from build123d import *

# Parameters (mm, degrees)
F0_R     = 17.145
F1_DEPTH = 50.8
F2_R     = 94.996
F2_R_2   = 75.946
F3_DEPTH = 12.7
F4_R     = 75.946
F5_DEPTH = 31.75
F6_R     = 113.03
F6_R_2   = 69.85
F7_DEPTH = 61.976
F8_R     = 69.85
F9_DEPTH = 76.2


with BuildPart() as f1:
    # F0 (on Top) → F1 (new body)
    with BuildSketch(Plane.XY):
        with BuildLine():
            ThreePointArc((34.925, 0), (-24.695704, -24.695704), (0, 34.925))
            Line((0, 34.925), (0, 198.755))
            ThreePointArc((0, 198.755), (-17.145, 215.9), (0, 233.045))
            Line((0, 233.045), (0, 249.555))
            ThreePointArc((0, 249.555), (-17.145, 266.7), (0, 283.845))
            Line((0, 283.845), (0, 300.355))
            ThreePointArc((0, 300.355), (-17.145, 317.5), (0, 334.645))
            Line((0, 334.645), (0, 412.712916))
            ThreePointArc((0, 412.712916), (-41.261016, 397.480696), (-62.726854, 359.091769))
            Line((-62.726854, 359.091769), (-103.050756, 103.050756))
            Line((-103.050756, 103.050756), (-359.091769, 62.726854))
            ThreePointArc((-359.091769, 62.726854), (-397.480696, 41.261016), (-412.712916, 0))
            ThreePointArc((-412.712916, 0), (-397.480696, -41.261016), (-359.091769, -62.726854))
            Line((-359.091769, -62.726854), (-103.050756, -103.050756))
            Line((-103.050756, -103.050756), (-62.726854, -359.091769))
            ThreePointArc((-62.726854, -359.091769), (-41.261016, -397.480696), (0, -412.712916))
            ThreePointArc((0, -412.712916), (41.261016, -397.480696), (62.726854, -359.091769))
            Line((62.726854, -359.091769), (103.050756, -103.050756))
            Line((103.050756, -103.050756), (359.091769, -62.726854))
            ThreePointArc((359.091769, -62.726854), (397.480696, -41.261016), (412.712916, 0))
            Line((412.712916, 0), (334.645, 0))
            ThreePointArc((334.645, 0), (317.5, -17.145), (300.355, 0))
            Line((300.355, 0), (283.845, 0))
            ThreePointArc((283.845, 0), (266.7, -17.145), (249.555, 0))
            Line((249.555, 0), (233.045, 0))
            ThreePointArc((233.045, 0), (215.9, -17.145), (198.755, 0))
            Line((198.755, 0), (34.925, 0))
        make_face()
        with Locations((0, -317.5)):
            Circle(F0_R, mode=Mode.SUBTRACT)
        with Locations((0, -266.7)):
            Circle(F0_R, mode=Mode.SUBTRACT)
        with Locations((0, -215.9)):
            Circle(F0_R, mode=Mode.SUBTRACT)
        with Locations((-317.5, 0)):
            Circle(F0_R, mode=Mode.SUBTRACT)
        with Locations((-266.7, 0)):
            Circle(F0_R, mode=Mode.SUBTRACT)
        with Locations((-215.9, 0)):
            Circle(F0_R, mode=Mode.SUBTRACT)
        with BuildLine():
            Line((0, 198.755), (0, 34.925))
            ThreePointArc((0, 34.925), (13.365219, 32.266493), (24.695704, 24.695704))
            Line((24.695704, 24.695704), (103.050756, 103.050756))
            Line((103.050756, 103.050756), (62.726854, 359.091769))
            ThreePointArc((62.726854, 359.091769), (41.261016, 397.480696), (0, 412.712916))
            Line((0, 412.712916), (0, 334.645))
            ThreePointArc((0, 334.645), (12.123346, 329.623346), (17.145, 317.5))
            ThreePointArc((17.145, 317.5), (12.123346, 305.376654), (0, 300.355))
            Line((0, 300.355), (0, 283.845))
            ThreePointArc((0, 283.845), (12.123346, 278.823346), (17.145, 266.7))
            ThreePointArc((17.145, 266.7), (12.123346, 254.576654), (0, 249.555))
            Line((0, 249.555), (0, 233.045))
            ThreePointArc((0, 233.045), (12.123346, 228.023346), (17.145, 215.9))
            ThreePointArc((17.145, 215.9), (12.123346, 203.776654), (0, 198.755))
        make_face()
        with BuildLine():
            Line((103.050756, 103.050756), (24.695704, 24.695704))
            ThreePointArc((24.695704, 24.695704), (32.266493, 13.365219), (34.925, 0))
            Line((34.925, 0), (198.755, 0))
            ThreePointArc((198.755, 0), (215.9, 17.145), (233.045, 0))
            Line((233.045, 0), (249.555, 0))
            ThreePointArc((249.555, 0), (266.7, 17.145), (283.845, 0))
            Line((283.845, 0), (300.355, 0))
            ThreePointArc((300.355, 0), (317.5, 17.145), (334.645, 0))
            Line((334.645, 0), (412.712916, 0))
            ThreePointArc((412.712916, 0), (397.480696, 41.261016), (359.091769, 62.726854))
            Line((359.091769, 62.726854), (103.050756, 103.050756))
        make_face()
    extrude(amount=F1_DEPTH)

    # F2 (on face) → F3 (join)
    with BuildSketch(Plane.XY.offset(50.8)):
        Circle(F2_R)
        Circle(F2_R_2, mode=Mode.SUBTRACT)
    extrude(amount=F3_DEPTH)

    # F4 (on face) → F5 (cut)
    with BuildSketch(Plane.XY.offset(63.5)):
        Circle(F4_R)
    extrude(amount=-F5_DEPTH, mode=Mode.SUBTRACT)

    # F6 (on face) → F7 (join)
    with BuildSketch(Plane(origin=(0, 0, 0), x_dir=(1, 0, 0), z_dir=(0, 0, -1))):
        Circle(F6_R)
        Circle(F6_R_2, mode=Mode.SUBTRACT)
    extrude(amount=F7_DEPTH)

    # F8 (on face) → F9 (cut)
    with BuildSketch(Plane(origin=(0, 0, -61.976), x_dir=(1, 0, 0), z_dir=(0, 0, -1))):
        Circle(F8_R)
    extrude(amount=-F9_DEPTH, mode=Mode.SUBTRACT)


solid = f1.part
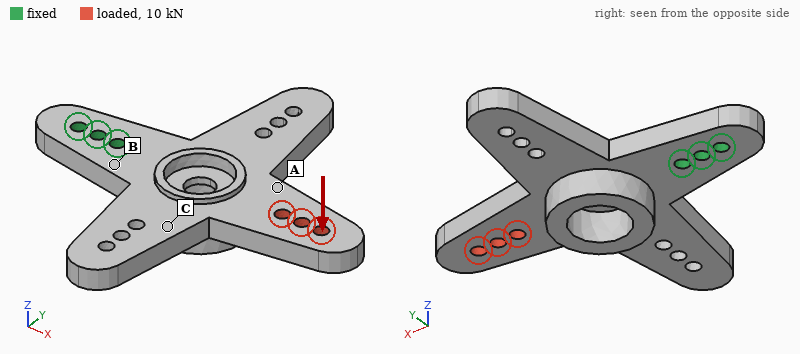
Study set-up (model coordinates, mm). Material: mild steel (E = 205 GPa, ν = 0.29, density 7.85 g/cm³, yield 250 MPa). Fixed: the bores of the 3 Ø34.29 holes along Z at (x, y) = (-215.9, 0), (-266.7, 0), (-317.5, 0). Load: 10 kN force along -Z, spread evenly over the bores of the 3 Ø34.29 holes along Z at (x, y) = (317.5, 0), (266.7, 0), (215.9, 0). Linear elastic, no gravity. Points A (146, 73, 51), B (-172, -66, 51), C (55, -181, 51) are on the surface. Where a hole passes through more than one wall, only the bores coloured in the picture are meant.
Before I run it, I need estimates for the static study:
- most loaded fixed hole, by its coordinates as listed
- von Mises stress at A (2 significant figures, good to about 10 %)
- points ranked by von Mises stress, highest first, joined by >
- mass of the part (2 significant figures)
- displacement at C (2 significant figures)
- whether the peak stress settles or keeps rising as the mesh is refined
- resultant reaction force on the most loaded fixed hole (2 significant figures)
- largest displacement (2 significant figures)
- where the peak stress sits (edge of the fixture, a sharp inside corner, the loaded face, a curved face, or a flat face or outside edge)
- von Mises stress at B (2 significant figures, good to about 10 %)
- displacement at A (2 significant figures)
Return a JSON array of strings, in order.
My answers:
["(-215.9, 0)", "15 MPa", "B > A > C", "96 kg", "0.30 mm", "keeps rising", "34 kN", "1.0 mm", "edge of the fixture", "47 MPa", "0.46 mm"]
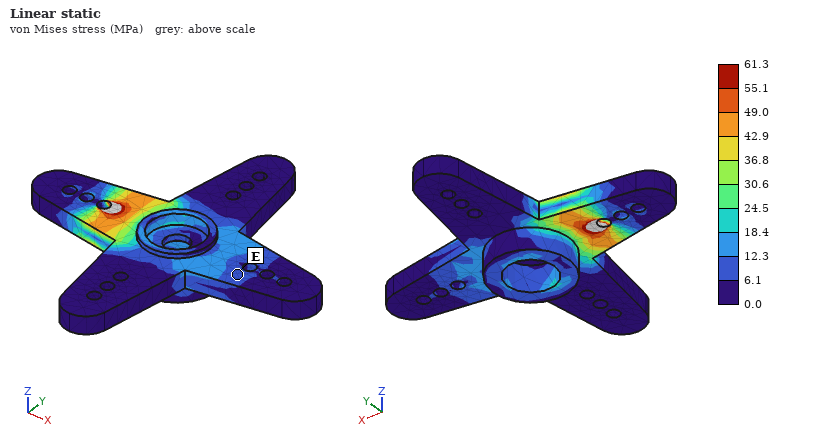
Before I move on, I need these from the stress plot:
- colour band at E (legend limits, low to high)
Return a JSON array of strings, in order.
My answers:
["6.1 to 12.3 MPa"]
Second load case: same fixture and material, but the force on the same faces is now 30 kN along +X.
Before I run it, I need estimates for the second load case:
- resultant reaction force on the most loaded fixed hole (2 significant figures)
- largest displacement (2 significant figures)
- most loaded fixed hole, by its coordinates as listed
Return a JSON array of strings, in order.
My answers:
["21 kN", "23 µm", "(-215.9, 0)"]
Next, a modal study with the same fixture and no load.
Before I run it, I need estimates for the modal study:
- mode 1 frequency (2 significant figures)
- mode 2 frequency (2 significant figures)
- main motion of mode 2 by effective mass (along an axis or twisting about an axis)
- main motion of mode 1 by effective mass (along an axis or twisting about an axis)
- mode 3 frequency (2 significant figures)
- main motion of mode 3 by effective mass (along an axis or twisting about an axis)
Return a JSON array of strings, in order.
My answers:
["120 Hz", "190 Hz", "twisting about X", "along Z", "250 Hz", "along Y"]
